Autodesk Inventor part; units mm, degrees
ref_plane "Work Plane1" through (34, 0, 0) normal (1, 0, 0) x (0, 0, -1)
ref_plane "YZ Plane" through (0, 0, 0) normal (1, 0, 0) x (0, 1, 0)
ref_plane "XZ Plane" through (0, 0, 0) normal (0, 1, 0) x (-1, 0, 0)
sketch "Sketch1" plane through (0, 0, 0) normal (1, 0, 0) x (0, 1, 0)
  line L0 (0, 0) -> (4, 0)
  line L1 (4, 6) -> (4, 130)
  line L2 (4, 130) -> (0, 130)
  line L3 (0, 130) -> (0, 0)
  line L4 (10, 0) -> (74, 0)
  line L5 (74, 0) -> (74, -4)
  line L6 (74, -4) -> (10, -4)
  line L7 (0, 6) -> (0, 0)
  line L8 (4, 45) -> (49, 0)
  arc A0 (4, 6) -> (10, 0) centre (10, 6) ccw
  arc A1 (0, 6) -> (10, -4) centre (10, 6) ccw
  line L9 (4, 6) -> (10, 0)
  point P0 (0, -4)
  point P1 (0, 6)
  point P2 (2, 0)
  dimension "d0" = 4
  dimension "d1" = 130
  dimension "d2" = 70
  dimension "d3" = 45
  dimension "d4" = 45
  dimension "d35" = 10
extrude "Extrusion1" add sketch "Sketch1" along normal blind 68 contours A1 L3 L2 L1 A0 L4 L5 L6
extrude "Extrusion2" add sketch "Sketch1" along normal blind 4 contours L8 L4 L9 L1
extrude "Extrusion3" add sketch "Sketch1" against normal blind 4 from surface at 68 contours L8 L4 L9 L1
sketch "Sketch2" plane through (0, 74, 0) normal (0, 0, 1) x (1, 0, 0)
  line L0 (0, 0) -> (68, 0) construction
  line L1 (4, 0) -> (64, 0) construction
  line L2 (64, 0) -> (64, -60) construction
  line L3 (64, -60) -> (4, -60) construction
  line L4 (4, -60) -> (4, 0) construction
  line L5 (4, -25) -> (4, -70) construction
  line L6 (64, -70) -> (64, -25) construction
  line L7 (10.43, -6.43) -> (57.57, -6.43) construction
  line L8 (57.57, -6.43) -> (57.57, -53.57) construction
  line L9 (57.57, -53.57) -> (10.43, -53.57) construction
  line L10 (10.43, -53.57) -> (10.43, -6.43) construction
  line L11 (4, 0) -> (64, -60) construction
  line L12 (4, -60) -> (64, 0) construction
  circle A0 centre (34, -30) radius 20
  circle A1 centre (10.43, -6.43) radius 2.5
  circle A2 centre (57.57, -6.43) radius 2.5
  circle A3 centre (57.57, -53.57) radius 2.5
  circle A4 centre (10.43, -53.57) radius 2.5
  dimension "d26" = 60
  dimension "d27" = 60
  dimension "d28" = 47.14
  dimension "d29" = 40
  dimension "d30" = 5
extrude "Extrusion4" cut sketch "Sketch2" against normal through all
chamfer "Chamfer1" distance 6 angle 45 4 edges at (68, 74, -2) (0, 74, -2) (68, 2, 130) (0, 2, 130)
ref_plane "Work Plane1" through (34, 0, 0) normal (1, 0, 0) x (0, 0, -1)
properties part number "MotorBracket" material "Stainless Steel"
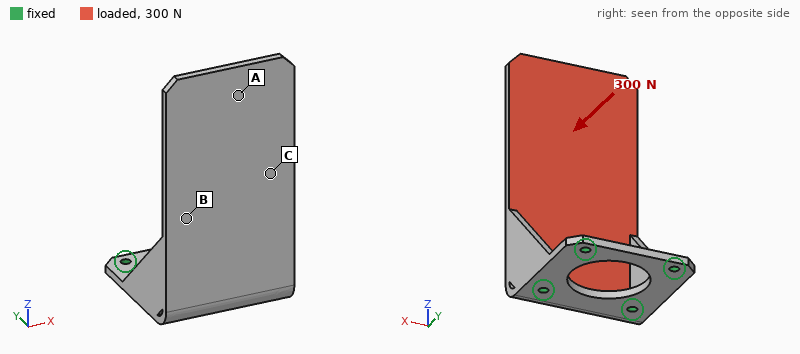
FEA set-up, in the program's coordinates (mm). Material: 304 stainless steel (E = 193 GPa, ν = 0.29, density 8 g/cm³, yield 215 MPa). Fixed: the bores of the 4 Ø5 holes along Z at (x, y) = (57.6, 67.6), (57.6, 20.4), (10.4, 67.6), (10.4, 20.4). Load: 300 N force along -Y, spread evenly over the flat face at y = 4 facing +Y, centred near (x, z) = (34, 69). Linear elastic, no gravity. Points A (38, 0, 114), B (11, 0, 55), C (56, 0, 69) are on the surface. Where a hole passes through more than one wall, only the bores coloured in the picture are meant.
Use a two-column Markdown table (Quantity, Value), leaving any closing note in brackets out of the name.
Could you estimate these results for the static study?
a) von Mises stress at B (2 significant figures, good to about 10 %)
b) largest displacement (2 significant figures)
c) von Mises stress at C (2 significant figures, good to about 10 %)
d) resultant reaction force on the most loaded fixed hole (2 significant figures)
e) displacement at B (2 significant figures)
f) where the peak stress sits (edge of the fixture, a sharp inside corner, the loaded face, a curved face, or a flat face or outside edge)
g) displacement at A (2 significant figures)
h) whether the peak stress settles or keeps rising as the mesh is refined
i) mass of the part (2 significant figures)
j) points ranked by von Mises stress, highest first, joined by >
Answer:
| Quantity | Value |
|---|---|
| von Mises stress at B | 46 MPa |
| largest displacement | 0.48 mm |
| von Mises stress at C | 30 MPa |
| resultant reaction force on the most loaded fixed hole | 240 N |
| displacement at B | 0.074 mm |
| where the peak stress sits | edge of the fixture |
| displacement at A | 0.39 mm |
| whether the peak stress settles or keeps rising as the mesh is refined | keeps rising |
| mass of the part | 460 g |
| points ranked by von Mises stress, highest first, joined by > | B > C > A |
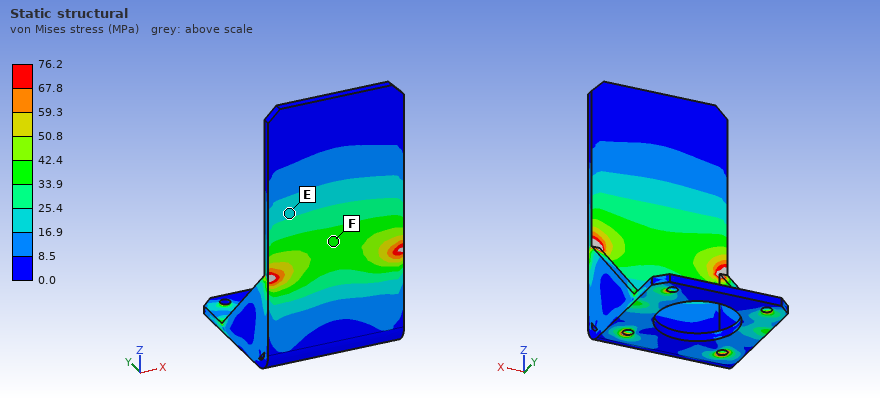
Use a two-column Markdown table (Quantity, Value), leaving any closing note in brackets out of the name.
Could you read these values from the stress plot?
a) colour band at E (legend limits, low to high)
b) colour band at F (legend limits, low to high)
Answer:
| Quantity | Value |
|---|---|
| colour band at E | 16.9 to 25.4 MPa |
| colour band at F | 33.9 to 42.4 MPa |
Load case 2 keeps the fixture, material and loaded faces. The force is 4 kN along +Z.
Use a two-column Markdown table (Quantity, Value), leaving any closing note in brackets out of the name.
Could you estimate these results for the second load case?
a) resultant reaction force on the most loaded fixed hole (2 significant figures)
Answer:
| Quantity | Value |
|---|---|
| resultant reaction force on the most loaded fixed hole | 2.5 kN |
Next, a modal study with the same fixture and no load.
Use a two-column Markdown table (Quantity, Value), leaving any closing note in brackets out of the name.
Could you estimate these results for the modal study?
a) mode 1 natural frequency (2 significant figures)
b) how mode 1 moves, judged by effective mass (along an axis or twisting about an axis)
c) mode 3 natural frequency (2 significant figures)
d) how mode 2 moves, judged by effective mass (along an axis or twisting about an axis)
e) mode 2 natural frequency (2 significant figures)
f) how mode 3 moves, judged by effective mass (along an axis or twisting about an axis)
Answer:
| Quantity | Value |
|---|---|
| mode 1 natural frequency | 310 Hz |
| how mode 1 moves, judged by effective mass | along Y |
| mode 3 natural frequency | 1300 Hz |
| how mode 2 moves, judged by effective mass | along X |
| mode 2 natural frequency | 890 Hz |
| how mode 3 moves, judged by effective mass | along X |
